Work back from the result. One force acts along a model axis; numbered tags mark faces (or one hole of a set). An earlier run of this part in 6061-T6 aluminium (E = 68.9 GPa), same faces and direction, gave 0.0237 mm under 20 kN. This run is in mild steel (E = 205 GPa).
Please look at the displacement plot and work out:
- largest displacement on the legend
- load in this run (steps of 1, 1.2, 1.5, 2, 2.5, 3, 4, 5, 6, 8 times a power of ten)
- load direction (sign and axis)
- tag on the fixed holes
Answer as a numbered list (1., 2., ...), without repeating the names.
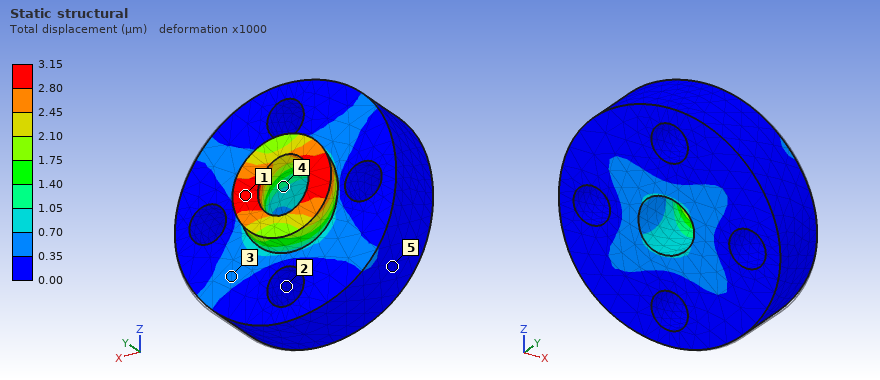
1. 3.15 µm
2. 8 kN
3. -X
4. 2
